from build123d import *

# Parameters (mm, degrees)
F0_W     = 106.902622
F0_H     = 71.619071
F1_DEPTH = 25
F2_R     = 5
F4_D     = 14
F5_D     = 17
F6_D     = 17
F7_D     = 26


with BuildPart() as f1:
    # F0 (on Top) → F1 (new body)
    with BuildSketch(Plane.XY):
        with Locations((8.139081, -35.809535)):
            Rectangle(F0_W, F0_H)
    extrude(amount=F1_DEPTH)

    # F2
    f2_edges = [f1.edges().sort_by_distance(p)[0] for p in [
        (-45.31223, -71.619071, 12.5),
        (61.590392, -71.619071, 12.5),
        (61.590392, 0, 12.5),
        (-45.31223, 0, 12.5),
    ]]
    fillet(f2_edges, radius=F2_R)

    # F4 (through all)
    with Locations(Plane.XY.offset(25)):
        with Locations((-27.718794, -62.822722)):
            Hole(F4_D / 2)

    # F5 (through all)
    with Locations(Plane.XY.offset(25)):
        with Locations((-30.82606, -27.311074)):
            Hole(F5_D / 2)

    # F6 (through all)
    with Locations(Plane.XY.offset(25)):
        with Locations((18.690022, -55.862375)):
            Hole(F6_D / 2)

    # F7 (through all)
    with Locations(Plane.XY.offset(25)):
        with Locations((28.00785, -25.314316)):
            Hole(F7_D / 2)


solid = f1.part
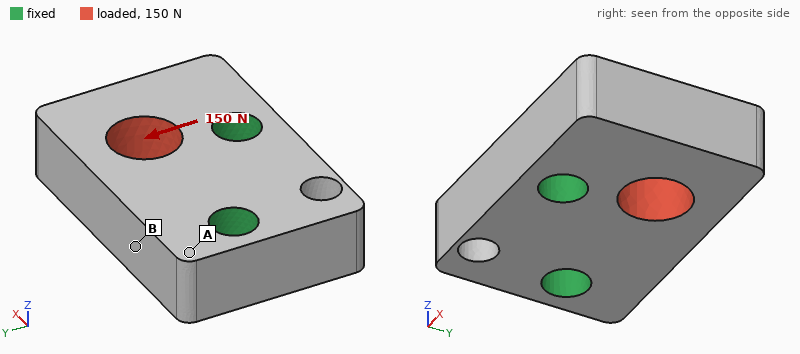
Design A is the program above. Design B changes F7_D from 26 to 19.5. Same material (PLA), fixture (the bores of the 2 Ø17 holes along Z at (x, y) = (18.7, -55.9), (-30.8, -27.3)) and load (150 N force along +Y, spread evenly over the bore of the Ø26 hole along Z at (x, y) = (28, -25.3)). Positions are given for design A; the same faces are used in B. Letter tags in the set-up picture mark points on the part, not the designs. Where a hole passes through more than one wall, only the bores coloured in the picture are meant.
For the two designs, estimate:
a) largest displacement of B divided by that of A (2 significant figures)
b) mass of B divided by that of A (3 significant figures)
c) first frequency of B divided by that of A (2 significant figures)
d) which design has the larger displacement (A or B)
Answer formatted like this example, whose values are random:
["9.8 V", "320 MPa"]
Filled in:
["0.75", "1.04", "1.0", "A"]
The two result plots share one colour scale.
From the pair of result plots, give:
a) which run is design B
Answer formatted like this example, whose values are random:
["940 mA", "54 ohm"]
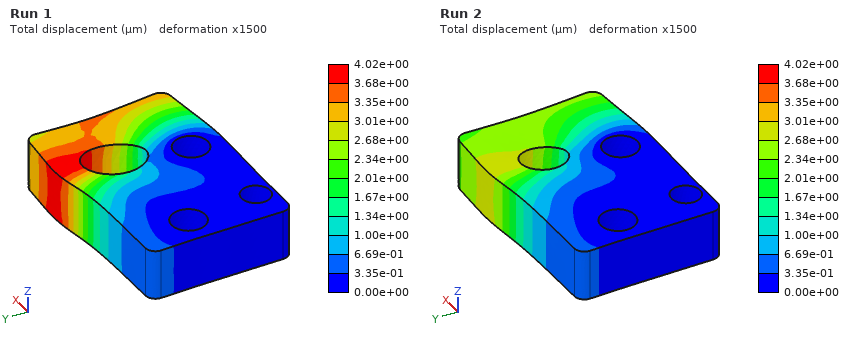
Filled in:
["Run 2"]
